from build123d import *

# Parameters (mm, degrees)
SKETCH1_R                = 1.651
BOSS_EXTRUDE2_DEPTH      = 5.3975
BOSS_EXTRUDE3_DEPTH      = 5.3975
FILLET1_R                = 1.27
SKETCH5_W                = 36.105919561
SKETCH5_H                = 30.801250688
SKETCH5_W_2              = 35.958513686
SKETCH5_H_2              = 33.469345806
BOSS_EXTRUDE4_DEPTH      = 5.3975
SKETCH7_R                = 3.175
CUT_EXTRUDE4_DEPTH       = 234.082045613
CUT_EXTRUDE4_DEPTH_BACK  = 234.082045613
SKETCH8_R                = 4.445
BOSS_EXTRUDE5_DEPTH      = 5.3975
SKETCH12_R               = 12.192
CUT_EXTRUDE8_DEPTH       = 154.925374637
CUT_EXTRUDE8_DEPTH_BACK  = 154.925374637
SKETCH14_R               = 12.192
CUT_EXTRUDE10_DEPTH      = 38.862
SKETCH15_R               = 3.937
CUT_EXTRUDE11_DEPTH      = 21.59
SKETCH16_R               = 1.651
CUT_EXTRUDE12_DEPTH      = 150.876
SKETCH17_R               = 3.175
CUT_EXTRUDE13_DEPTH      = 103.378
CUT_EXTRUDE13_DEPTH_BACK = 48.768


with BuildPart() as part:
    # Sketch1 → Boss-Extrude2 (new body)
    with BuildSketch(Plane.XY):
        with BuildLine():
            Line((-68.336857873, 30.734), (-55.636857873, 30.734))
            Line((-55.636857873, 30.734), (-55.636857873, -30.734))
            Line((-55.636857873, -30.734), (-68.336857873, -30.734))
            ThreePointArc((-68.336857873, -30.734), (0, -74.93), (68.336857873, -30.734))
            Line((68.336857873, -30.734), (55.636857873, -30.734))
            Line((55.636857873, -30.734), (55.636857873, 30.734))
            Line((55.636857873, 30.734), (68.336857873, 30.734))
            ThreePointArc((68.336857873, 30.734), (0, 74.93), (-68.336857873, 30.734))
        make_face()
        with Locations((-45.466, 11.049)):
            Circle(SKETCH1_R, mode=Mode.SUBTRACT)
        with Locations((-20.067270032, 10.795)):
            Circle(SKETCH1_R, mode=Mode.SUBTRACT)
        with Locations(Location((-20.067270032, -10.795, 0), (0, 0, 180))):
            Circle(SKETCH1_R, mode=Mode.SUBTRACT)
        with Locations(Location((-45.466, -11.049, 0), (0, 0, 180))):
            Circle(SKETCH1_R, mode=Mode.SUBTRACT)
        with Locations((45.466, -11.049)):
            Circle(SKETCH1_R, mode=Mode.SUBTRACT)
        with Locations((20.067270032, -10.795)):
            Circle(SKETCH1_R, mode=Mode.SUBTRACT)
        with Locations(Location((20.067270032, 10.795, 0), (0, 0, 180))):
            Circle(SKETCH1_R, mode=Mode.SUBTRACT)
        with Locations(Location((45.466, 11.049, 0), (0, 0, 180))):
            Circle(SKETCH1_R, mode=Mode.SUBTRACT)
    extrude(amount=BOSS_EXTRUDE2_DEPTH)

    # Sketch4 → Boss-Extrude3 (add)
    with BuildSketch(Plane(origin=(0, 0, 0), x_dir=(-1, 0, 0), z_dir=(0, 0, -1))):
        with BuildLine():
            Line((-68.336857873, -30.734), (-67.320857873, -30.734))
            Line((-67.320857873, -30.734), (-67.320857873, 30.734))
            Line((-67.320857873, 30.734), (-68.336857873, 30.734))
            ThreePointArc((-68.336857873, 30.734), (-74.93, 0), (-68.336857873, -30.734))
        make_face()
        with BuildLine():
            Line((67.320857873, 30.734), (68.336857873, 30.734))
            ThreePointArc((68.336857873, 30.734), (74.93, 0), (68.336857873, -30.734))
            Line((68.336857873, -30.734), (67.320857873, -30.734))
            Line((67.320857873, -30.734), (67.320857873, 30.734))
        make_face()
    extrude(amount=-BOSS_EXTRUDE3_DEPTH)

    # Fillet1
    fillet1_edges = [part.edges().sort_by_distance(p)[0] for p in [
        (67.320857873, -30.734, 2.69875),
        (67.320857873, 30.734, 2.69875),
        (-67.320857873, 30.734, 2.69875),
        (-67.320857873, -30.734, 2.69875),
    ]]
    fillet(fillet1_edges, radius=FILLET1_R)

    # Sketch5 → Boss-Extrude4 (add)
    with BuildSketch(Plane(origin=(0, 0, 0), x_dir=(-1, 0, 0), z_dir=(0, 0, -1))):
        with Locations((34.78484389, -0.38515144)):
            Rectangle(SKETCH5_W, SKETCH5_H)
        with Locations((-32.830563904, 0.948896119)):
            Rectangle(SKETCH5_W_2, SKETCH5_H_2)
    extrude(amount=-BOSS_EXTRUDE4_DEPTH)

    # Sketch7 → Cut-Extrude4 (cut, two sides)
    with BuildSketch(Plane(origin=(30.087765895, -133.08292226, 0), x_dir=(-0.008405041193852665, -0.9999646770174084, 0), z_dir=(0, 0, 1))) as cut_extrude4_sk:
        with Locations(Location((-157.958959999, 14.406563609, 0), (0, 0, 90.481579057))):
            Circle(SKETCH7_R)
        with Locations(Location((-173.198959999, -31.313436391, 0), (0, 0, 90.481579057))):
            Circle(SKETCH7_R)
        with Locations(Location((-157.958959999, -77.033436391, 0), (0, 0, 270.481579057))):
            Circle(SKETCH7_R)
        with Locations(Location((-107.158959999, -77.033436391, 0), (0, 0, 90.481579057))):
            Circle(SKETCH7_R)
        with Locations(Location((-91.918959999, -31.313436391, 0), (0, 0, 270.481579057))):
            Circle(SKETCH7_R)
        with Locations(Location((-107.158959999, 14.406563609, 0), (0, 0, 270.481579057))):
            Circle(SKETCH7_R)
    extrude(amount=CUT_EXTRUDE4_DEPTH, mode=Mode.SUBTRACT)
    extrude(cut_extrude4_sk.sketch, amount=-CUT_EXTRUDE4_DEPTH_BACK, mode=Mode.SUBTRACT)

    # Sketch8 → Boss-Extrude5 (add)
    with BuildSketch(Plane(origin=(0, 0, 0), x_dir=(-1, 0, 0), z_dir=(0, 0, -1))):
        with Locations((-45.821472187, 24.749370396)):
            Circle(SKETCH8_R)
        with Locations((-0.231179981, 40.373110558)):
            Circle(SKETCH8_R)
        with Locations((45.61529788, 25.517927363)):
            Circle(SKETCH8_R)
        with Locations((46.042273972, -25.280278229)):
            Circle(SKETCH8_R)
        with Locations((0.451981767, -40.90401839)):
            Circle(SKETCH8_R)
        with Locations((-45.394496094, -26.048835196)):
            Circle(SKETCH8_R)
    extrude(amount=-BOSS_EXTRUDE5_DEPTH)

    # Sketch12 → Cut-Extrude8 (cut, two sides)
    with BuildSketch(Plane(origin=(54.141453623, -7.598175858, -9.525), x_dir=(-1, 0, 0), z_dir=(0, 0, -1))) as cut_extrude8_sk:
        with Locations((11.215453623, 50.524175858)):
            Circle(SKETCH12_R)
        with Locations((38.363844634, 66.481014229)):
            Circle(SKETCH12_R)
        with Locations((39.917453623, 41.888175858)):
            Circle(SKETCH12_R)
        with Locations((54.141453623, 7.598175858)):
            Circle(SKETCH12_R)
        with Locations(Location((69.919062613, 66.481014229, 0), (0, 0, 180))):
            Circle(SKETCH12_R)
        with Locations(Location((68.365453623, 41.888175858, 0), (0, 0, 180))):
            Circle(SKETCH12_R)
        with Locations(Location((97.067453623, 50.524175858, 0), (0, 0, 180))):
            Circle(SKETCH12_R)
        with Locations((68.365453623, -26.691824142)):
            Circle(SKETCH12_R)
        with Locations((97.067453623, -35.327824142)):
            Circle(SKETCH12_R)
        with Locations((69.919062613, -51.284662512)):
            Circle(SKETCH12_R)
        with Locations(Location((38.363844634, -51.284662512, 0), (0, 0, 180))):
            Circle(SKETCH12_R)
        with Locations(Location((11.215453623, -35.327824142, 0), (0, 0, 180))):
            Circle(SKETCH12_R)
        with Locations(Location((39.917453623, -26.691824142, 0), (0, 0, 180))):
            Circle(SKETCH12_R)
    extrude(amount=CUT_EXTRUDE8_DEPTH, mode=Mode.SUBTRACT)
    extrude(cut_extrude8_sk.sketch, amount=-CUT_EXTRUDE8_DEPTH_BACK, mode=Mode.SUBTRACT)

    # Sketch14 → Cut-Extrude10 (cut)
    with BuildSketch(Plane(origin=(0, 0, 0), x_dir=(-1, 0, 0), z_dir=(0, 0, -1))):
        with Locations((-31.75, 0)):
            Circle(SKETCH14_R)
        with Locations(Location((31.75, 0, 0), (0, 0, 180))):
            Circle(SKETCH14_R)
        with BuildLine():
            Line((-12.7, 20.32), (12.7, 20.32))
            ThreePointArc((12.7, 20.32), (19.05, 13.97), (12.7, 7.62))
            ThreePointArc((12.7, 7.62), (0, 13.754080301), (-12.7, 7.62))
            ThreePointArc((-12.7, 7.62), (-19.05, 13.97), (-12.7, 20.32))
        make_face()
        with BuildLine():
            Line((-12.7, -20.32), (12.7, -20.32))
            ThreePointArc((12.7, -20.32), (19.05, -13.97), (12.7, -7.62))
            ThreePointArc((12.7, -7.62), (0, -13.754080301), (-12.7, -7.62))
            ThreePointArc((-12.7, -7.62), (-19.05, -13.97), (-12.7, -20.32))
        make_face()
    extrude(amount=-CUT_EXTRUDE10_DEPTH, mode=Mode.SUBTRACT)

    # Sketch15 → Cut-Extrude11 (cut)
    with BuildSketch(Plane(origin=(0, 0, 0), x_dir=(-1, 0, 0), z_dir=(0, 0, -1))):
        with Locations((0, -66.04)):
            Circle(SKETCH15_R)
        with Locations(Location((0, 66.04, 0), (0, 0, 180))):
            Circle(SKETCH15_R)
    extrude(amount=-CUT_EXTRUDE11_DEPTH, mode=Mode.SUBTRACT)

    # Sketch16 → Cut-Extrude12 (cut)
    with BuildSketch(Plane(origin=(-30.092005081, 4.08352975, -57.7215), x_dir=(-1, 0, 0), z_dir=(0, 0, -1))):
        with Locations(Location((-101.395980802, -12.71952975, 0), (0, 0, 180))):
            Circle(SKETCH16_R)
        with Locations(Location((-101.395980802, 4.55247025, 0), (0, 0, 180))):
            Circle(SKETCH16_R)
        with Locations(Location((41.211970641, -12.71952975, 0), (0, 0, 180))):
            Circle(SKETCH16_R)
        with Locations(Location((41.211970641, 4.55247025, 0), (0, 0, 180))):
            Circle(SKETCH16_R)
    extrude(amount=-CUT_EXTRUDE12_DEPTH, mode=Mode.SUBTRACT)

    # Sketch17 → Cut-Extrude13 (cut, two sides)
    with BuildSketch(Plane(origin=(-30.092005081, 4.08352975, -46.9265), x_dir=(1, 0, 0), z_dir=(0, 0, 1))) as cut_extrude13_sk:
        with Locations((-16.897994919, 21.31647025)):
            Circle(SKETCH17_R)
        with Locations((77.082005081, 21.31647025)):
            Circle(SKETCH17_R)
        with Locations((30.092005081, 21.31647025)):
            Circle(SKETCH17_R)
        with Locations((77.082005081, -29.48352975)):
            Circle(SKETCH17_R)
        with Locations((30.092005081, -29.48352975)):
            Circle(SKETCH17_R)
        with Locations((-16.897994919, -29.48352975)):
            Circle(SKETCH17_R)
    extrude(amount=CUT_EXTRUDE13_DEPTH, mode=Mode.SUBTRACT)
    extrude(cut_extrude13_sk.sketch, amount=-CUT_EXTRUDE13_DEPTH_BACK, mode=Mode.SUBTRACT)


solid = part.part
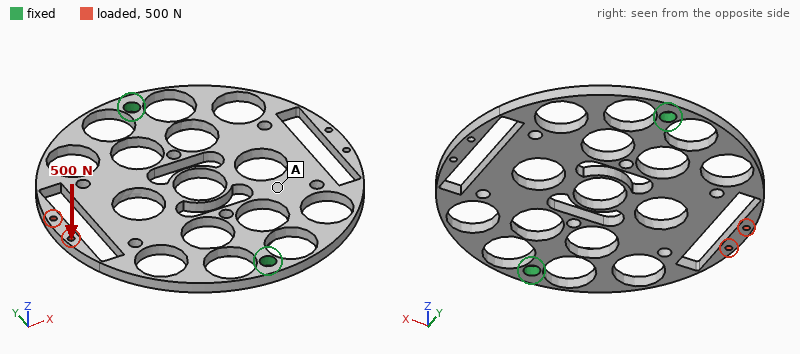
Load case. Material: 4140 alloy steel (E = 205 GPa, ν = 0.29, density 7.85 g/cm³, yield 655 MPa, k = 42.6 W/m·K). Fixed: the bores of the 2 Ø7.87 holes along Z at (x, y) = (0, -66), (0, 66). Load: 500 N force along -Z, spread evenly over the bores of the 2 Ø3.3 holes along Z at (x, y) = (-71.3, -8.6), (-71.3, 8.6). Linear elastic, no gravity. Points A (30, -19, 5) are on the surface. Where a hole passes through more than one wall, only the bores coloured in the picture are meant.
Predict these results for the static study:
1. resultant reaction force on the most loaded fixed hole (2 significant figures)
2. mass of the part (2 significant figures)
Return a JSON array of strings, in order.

["250 N", "350 g"]
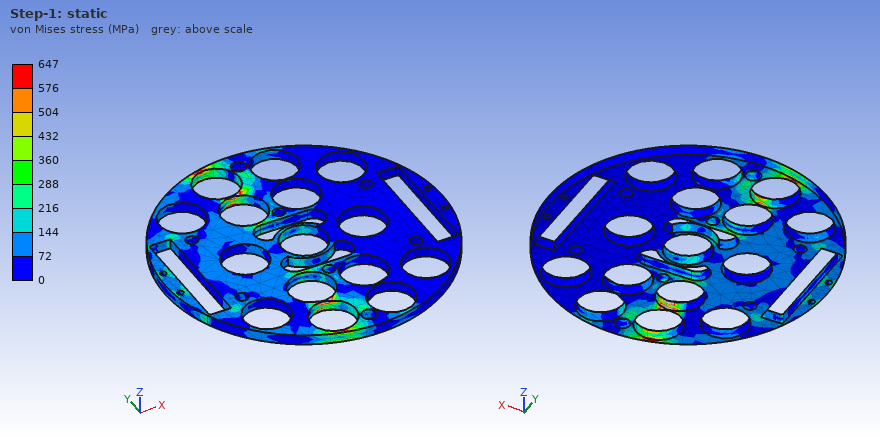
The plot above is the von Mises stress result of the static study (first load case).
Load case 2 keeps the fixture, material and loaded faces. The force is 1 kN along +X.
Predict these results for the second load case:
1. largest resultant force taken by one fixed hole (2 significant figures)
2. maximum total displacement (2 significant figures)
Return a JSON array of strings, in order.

["510 N", "0.12 mm"]
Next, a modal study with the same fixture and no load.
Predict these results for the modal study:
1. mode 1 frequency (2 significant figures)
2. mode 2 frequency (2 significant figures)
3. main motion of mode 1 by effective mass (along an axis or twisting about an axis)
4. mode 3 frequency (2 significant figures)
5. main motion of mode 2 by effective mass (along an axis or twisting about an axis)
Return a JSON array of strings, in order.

["380 Hz", "500 Hz", "twisting about Y", "1400 Hz", "along Z"]
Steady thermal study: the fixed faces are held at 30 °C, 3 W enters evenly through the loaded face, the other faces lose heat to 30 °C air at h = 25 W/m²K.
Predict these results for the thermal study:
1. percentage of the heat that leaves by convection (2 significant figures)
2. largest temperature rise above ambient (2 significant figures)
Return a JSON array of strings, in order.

["90 %", "46 K"]
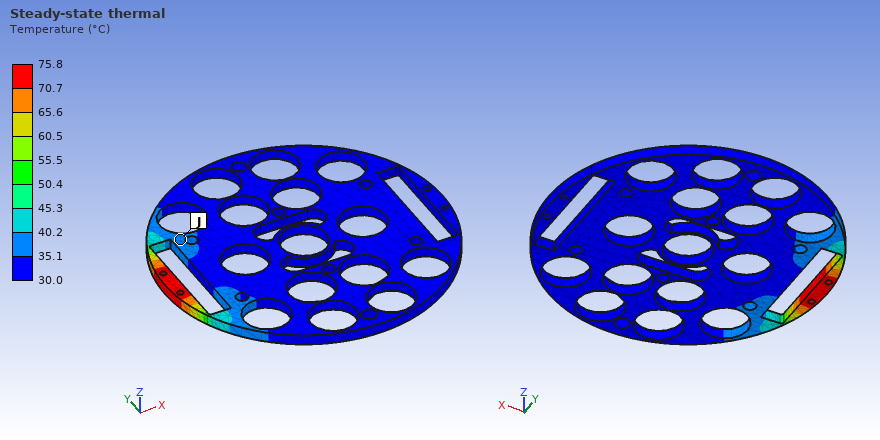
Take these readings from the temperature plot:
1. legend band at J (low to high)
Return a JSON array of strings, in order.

["35.1 to 40.2 °C"]
